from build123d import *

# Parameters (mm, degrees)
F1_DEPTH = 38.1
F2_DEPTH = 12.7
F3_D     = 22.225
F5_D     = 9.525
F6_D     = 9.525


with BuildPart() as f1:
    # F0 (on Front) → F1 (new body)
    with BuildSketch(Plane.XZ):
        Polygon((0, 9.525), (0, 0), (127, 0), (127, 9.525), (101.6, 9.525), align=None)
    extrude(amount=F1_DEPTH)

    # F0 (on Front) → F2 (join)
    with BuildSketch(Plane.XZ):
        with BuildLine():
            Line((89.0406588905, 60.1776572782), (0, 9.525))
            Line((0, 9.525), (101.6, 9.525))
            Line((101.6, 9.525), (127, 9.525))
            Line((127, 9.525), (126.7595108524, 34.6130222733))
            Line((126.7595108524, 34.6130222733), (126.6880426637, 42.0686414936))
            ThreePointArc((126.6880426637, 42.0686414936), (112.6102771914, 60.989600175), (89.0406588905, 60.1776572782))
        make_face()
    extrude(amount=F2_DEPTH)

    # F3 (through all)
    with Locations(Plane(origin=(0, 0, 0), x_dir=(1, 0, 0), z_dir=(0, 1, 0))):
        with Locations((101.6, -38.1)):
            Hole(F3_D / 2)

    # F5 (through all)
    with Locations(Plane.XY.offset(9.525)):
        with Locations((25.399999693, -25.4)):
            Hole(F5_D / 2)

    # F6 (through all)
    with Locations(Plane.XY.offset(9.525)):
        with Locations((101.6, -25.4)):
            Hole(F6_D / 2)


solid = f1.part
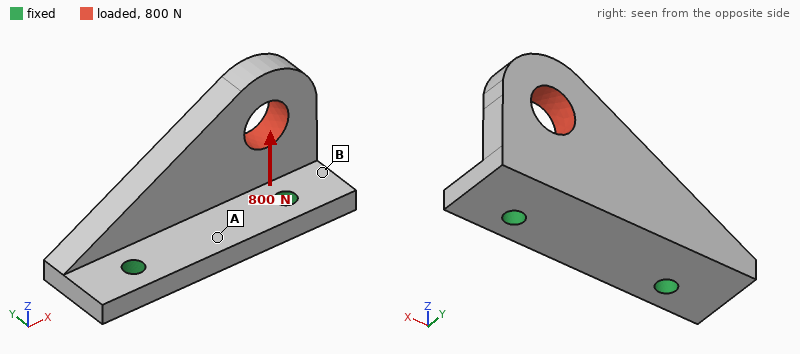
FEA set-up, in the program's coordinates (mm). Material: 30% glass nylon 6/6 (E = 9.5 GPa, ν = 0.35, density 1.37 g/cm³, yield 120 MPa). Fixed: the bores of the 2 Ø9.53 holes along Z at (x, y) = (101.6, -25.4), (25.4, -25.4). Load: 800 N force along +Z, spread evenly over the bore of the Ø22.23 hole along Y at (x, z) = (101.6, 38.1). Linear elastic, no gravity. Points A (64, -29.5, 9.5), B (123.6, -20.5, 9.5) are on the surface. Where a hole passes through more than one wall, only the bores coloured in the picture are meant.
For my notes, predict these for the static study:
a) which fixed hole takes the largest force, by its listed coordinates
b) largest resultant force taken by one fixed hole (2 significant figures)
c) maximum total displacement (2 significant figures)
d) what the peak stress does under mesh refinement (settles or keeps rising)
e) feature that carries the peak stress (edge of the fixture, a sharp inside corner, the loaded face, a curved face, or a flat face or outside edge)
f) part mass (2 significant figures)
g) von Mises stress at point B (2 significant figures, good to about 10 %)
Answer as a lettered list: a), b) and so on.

a) (101.6, -25.4)
b) 770 N
c) 0.19 mm
d) keeps rising
e) edge of the fixture
f) 130 g
g) 4.2 MPa
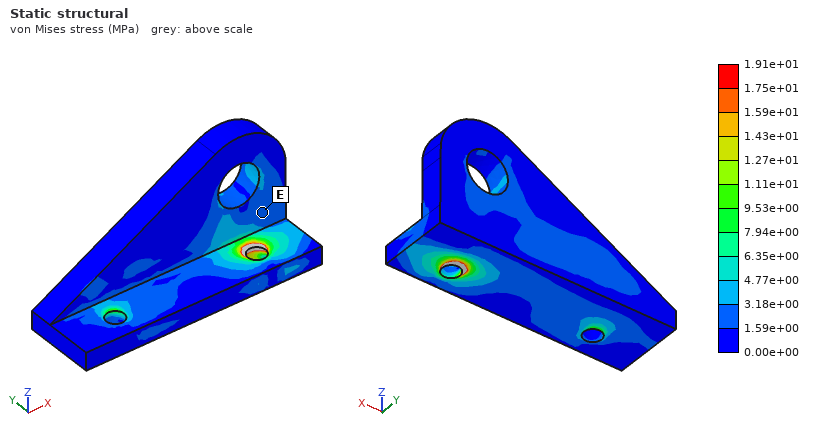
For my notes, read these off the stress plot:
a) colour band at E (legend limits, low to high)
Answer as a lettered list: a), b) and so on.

a) 1.59e+00 to 3.18e+00 MPa
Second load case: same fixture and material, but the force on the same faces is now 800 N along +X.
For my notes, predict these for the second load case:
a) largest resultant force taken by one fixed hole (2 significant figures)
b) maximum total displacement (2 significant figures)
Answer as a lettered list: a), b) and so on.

a) 550 N
b) 66 µm
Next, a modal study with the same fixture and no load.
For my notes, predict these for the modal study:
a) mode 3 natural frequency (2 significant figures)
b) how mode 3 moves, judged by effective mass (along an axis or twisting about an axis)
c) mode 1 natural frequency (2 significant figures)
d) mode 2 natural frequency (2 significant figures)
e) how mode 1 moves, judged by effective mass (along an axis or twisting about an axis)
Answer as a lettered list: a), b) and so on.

a) 3300 Hz
b) along Z
c) 1100 Hz
d) 2600 Hz
e) along Y
